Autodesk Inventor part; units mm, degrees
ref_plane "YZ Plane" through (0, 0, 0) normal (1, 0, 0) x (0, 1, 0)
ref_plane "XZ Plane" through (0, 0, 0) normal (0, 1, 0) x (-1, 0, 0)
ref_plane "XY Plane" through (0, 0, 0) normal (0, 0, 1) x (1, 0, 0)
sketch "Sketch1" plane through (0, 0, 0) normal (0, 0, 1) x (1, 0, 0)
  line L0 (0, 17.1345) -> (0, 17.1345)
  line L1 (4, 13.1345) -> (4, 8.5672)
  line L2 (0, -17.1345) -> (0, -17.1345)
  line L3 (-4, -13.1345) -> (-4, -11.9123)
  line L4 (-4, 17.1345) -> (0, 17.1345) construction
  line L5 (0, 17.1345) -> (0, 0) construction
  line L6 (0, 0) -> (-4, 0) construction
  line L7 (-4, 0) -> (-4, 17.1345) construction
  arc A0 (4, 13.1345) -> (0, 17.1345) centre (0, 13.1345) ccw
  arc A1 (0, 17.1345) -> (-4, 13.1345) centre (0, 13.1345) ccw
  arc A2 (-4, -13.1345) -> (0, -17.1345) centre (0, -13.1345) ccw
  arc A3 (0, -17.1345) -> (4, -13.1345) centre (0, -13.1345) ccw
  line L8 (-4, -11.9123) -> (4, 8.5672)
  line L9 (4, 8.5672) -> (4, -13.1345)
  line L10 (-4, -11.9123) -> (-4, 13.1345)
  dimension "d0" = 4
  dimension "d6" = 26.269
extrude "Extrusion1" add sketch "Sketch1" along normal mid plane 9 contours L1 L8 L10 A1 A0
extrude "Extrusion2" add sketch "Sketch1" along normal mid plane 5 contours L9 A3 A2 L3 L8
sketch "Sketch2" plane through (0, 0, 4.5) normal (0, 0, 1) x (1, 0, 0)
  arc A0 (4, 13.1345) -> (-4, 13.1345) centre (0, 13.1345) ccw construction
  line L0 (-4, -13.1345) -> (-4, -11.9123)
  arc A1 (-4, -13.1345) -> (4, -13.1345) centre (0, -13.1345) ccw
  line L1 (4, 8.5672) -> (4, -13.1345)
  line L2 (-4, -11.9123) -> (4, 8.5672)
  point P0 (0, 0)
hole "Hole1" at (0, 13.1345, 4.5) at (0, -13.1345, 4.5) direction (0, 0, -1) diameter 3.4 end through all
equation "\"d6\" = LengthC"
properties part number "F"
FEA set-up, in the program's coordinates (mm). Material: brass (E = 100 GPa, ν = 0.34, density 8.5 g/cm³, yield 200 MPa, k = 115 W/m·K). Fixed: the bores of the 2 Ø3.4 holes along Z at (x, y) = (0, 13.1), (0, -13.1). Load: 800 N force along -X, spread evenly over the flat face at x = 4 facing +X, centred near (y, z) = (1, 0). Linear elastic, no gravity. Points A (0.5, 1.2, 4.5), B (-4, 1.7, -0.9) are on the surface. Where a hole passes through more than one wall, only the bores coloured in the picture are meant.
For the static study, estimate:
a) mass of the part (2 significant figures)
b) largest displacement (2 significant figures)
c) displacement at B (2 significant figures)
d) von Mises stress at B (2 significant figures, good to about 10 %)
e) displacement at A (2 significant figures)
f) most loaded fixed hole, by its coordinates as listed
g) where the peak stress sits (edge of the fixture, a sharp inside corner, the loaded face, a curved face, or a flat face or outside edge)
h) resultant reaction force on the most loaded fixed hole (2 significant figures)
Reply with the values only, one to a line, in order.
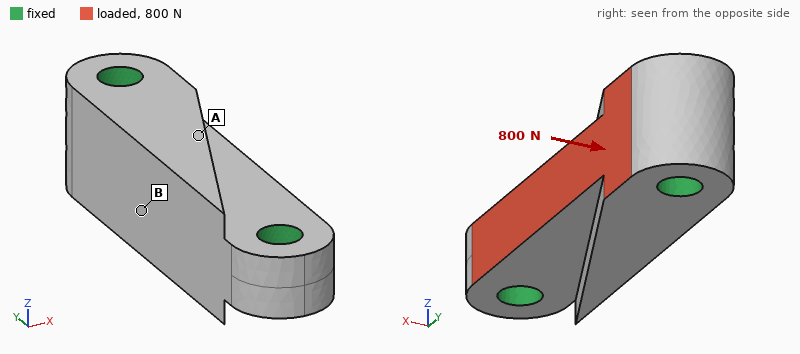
15 g
2.8 µm
2.5 µm
11 MPa
2.6 µm
(0, 13.1)
edge of the fixture
460 N
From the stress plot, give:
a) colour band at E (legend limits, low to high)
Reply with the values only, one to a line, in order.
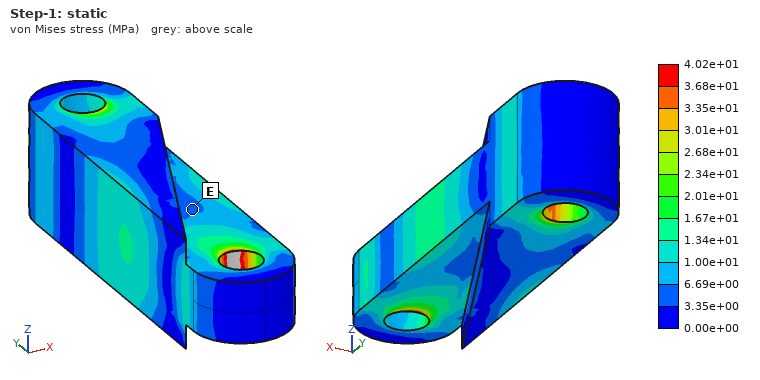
3.35e+00 to 6.69e+00 MPa
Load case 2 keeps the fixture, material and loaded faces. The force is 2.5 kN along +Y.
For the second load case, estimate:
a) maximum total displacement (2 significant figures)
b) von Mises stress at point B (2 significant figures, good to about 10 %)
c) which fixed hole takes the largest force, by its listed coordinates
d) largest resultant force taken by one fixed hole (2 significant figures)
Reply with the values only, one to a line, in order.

2.7 µm
5.3 MPa
(0, 13.1)
1.5 kN
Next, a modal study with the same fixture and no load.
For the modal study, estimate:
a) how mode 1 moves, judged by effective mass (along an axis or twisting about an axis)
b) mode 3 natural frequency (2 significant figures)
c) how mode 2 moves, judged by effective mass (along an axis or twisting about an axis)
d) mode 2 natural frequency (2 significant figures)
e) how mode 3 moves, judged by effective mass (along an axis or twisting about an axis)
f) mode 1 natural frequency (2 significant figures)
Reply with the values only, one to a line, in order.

along X
36 kHz
along Z
28 kHz
twisting about Y
25 kHz
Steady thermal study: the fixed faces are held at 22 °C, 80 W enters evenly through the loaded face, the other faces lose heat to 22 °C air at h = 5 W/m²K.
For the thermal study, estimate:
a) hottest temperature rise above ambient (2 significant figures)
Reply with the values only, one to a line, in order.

47 K
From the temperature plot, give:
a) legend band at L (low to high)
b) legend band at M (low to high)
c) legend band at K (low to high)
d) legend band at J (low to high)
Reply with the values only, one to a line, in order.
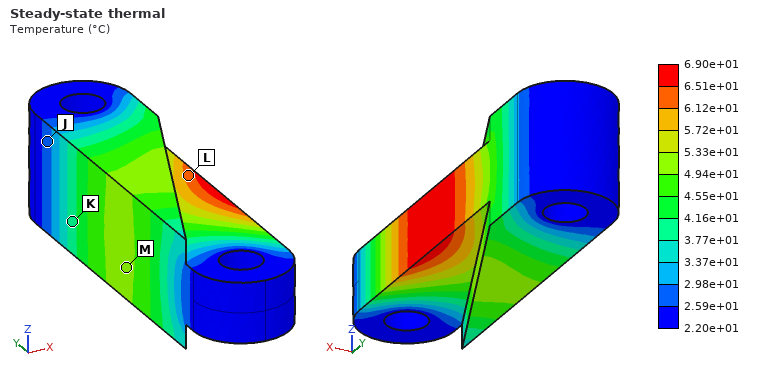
6.12e+01 to 6.51e+01 °C
4.94e+01 to 5.33e+01 °C
3.77e+01 to 4.16e+01 °C
2.59e+01 to 2.98e+01 °C
